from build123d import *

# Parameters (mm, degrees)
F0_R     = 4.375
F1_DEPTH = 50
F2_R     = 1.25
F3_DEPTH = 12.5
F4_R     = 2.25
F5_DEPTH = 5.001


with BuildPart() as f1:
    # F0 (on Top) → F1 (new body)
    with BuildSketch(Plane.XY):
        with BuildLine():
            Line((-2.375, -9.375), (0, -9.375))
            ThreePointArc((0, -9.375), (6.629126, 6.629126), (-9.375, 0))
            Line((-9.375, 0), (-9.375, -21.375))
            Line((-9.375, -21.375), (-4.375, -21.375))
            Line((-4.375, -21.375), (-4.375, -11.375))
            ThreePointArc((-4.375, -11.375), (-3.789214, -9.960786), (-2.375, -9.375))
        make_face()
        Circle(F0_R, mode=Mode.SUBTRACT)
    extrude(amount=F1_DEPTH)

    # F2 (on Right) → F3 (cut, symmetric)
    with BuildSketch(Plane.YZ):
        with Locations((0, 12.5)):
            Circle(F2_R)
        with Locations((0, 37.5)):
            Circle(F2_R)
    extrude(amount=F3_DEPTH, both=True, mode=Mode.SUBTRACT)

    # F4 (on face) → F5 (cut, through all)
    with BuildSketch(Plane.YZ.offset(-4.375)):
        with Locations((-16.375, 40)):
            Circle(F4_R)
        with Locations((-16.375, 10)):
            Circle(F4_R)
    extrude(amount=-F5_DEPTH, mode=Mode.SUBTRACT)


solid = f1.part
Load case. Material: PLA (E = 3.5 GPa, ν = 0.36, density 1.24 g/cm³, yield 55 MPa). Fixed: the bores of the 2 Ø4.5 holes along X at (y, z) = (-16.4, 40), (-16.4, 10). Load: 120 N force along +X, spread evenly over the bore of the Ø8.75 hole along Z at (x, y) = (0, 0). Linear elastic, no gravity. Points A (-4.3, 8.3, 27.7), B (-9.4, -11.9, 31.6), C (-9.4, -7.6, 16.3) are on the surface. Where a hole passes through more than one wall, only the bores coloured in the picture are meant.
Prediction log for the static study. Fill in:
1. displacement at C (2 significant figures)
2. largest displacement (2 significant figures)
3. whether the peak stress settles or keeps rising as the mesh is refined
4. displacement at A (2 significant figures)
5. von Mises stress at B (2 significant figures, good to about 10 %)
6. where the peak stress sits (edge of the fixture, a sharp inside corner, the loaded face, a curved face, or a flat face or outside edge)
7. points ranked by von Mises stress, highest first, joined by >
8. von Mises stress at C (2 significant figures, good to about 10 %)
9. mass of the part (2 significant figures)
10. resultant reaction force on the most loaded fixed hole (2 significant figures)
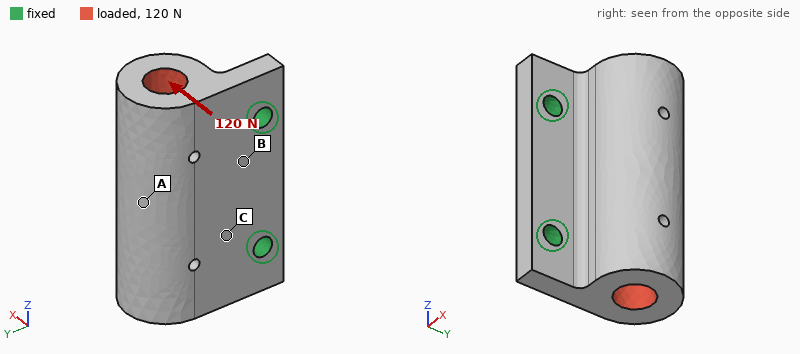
0.050 mm
0.19 mm
keeps rising
0.17 mm
4.1 MPa
edge of the fixture
B > C > A
2.5 MPa
18 g
60 N
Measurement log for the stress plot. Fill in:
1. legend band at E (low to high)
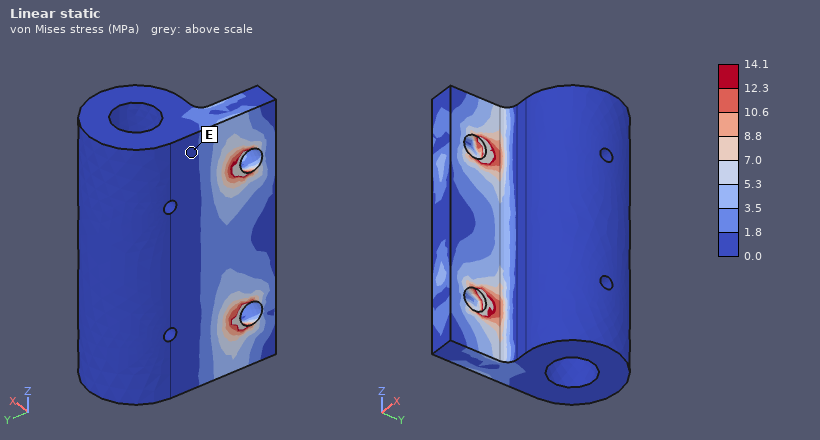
0.0 to 1.8 MPa
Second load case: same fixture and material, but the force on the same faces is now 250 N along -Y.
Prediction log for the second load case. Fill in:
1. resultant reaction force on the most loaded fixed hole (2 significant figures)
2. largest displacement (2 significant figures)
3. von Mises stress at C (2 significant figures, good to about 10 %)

130 N
0.22 mm
3.0 MPa
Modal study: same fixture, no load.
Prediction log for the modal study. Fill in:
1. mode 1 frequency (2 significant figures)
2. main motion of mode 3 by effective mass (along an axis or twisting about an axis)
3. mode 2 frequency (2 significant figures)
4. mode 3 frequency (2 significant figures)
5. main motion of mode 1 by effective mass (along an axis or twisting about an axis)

1200 Hz
along Z
3400 Hz
4600 Hz
along X
